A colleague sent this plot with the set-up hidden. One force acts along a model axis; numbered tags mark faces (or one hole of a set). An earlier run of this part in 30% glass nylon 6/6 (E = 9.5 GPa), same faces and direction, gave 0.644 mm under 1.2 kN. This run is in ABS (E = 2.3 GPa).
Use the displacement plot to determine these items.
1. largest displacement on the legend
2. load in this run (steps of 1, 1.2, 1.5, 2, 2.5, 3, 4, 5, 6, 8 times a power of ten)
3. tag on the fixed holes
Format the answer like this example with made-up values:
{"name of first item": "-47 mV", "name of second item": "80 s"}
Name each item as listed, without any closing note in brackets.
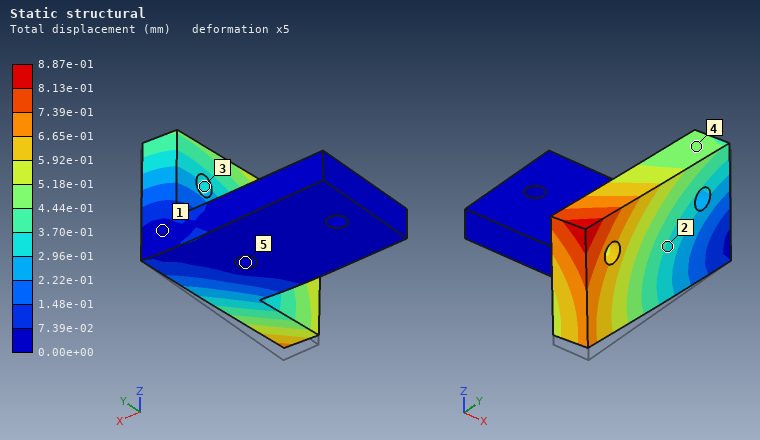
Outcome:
{"largest displacement on the legend": "8.87e-01 mm", "load in this run": "400 N", "tag on the fixed holes": "5"}
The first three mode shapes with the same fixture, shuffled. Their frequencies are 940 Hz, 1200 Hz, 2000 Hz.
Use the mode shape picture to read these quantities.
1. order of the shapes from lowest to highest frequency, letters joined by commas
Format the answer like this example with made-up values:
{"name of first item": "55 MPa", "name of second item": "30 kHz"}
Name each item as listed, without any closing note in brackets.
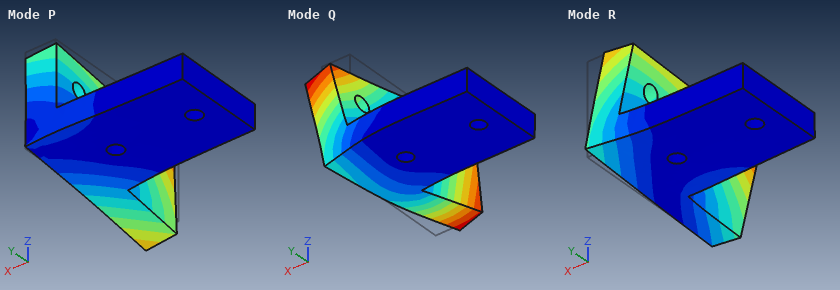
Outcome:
{"order of the shapes from lowest to highest frequency, letters joined by commas": "P, R, Q"}
